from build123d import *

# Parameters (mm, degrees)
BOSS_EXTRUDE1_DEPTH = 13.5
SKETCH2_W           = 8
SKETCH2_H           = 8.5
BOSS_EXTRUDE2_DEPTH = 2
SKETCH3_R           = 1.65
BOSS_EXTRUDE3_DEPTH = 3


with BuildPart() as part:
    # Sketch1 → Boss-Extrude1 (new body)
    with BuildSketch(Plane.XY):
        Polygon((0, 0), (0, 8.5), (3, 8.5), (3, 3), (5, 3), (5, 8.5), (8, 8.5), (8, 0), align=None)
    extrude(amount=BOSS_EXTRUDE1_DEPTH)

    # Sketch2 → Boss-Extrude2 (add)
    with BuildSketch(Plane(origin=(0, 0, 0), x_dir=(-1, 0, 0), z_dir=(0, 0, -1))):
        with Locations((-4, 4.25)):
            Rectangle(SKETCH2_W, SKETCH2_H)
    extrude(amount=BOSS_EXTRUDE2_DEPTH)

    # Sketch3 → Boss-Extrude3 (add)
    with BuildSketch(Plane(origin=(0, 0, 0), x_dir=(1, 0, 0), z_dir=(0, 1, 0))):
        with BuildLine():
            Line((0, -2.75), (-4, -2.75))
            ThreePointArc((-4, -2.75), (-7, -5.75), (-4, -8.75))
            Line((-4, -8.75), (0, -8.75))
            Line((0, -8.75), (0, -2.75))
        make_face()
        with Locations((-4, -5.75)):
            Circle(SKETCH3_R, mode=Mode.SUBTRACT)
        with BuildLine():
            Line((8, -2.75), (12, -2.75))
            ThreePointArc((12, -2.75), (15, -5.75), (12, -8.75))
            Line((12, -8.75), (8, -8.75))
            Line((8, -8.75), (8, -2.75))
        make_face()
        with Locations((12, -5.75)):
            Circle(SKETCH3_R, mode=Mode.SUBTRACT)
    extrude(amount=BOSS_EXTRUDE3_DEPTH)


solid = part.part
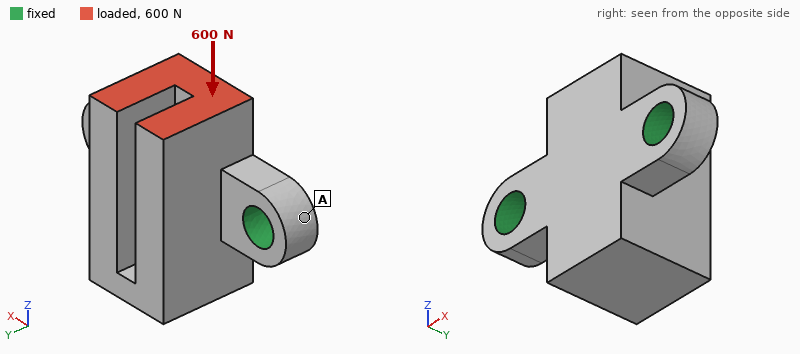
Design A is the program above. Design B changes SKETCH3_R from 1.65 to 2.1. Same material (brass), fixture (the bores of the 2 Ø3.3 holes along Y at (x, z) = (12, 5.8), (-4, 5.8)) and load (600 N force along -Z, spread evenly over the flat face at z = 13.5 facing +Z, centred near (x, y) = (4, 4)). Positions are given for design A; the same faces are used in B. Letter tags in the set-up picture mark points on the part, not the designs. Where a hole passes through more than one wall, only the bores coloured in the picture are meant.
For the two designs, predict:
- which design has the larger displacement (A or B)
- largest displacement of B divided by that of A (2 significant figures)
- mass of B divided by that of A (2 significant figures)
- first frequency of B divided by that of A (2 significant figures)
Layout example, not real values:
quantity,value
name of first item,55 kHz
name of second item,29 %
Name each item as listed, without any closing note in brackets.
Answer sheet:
quantity,value
which design has the larger displacement,A
largest displacement of B divided by that of A,0.83
mass of B divided by that of A,0.97
first frequency of B divided by that of A,1.1
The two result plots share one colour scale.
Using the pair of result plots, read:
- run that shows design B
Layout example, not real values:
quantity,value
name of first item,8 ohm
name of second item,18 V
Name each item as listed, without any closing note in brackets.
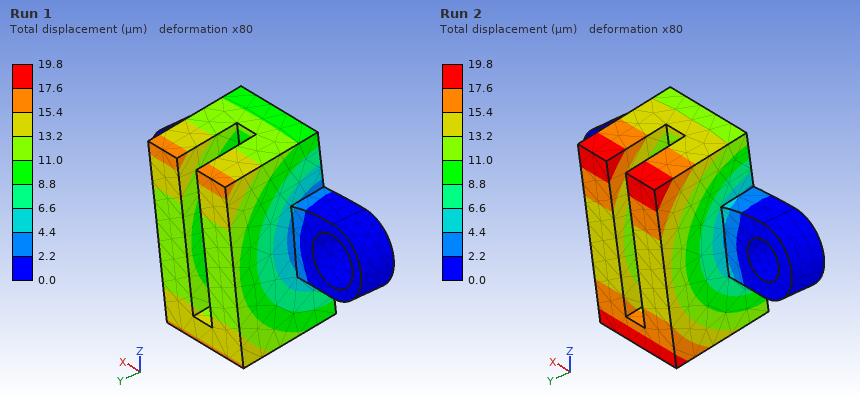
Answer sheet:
quantity,value
run that shows design B,Run 1
